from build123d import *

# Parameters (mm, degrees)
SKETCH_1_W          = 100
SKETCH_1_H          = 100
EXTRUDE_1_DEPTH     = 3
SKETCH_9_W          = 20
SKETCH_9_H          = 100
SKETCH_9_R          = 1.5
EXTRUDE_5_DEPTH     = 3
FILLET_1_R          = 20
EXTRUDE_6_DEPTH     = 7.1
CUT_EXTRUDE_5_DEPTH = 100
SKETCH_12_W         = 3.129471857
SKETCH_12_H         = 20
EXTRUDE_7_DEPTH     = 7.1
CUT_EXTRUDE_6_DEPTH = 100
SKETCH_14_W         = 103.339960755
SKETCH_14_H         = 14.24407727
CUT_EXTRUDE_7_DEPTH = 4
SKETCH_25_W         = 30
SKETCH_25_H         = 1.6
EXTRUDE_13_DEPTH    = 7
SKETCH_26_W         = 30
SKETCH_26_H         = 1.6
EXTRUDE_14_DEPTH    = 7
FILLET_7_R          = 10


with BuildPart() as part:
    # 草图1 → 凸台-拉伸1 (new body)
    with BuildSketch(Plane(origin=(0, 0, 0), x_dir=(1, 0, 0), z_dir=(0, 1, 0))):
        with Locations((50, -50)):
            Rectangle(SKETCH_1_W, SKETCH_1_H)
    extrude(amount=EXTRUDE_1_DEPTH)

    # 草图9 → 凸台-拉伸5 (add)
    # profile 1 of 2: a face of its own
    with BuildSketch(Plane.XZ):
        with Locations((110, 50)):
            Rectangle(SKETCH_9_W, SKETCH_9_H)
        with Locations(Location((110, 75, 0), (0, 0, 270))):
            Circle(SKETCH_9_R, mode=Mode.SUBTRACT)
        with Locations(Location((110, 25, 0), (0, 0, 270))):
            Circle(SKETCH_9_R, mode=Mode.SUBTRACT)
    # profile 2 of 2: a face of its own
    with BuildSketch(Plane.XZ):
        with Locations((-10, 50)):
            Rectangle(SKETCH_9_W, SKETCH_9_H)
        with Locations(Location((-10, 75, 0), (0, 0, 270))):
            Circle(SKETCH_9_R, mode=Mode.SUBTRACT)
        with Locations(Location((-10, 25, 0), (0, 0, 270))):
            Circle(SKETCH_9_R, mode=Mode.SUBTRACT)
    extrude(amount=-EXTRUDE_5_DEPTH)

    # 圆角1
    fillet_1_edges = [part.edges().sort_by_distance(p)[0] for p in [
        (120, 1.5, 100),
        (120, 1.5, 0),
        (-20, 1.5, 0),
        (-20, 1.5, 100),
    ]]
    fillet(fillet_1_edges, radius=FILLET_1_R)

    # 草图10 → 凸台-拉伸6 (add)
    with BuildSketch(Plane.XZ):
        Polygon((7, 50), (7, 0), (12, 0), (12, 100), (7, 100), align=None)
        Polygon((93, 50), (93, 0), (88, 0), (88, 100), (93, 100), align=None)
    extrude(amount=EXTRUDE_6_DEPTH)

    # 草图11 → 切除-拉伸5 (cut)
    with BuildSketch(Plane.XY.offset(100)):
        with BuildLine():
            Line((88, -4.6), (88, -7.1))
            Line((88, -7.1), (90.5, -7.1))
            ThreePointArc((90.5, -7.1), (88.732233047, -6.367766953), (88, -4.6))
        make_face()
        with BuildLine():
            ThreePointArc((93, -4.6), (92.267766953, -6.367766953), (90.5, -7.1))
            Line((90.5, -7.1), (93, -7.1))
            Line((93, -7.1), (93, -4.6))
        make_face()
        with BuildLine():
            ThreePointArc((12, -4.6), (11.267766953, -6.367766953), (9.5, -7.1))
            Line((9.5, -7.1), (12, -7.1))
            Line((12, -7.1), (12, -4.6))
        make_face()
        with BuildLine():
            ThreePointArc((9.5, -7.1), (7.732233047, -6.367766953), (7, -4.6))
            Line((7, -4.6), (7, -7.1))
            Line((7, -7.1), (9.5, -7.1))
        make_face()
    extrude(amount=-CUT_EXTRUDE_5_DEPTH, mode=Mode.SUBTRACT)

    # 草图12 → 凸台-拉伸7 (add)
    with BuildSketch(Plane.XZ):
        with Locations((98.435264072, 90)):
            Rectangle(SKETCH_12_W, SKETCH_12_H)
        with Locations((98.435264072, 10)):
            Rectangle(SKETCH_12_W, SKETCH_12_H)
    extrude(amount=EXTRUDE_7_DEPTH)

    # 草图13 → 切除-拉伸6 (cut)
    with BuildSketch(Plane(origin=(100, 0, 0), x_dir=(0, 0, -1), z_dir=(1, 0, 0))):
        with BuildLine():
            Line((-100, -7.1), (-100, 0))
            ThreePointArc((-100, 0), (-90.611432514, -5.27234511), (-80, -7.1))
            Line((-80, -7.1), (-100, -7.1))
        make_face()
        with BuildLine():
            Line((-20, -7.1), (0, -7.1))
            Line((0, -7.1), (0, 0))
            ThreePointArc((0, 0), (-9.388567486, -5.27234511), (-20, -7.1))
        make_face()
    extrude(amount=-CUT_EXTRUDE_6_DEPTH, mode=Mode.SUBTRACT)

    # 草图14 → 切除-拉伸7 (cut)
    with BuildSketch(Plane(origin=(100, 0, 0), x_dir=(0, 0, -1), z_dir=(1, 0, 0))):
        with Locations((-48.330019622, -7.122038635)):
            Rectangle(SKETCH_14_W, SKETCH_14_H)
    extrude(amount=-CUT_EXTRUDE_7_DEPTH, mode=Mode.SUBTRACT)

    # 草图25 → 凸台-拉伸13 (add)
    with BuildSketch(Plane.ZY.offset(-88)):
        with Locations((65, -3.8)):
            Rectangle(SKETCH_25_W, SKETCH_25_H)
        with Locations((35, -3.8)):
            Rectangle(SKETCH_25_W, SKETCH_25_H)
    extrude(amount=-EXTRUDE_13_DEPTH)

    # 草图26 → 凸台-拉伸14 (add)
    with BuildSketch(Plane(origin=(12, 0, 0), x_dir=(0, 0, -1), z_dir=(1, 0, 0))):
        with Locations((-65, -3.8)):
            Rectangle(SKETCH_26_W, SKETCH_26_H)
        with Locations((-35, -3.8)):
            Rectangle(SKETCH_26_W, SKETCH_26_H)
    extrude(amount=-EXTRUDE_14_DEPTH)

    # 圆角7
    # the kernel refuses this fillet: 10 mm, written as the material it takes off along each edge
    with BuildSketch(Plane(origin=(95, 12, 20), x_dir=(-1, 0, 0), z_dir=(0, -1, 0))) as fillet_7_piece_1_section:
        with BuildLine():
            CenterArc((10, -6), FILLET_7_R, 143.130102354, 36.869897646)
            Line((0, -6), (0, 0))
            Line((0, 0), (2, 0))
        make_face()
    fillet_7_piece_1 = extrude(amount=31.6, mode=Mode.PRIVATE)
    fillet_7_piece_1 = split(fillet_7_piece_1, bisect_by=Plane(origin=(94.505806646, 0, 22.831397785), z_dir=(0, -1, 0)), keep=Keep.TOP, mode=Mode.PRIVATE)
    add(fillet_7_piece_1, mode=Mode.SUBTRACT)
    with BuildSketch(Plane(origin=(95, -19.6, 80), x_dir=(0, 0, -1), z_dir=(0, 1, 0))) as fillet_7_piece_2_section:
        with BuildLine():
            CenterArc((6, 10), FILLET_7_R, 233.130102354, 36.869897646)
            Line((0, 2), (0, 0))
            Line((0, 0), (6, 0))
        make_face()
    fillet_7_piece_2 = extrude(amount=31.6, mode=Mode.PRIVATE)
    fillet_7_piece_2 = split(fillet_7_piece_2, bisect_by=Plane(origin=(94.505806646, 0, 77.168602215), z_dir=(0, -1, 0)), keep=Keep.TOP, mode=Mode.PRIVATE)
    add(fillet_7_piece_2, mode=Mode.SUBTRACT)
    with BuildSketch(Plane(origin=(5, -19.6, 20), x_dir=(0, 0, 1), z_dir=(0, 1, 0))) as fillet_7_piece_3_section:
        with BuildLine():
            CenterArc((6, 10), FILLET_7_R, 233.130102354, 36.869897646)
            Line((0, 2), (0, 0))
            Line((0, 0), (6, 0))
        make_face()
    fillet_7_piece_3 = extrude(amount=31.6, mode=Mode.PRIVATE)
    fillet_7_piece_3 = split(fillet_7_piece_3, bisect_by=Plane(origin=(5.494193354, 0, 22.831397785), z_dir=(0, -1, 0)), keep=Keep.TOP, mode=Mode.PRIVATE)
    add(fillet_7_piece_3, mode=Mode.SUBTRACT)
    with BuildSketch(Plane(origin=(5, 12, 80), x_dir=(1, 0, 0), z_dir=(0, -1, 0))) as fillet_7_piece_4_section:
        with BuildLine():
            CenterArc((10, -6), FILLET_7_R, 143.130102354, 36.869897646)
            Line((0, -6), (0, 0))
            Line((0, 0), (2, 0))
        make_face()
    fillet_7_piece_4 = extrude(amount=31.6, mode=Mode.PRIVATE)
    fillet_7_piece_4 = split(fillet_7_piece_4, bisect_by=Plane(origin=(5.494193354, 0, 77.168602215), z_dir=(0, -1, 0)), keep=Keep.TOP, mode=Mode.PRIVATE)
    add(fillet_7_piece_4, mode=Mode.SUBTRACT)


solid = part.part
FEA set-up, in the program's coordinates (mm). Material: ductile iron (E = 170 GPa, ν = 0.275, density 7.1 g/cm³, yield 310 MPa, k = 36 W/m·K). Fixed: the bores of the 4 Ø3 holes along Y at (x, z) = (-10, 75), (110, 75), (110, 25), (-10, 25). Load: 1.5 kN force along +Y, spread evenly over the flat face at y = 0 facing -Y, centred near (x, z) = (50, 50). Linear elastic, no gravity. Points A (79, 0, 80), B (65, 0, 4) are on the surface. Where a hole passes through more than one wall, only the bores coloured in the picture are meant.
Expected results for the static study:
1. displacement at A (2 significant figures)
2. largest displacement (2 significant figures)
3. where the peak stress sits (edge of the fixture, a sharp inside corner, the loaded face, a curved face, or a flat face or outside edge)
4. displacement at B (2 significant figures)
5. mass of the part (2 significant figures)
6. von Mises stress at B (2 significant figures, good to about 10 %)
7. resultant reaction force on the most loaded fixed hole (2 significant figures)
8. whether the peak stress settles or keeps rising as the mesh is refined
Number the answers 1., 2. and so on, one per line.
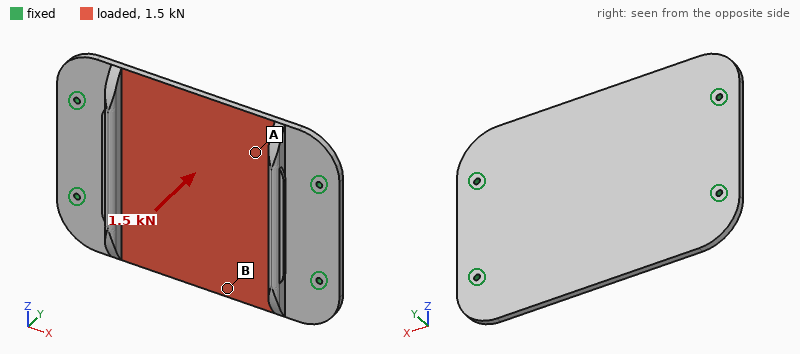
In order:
1. 0.22 mm
2. 0.36 mm
3. edge of the fixture
4. 0.31 mm
5. 330 g
6. 74 MPa
7. 380 N
8. keeps rising
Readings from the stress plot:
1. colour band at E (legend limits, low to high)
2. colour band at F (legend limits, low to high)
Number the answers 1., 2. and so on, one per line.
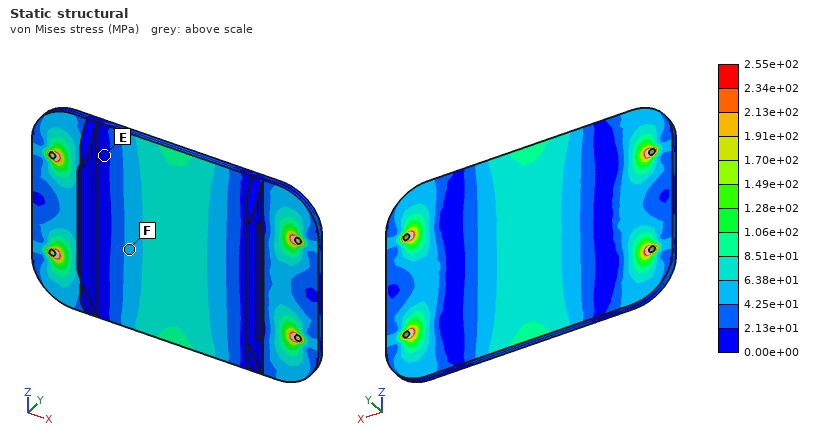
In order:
1. 0.00e+00 to 2.13e+01 MPa
2. 4.25e+01 to 6.38e+01 MPa
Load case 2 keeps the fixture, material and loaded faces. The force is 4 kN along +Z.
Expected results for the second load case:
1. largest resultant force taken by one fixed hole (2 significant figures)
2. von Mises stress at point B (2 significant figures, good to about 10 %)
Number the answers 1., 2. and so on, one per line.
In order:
1. 1.1 kN
2. 7.8 MPa
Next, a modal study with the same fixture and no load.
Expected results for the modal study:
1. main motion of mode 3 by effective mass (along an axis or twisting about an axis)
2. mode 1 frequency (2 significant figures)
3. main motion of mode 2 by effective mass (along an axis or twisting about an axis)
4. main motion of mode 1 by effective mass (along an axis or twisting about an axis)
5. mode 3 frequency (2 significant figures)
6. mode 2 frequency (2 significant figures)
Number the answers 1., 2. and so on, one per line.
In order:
1. twisting about Z
2. 870 Hz
3. twisting about X
4. along Y
5. 2300 Hz
6. 1200 Hz
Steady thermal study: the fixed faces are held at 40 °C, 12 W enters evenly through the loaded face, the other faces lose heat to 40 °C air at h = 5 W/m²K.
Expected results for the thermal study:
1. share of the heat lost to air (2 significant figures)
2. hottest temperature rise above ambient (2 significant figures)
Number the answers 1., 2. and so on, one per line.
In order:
1. 15 %
2. 26 K
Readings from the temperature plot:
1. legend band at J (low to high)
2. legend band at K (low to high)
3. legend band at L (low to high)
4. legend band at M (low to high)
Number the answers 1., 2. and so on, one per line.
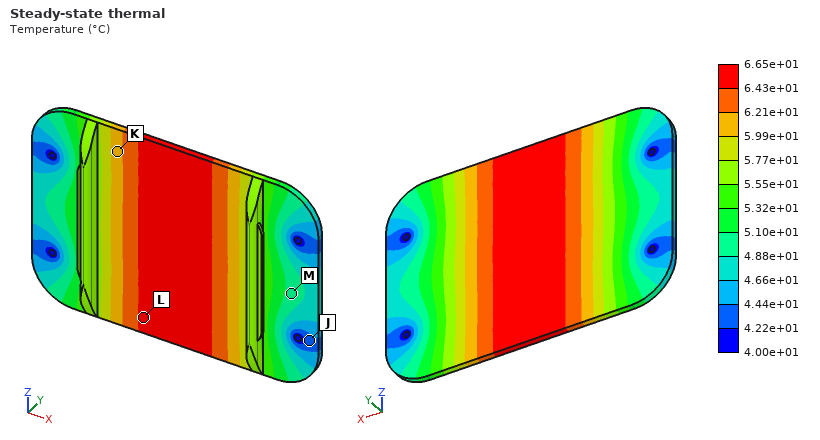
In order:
1. 4.22e+01 to 4.44e+01 °C
2. 5.99e+01 to 6.21e+01 °C
3. 6.43e+01 to 6.65e+01 °C
4. 4.88e+01 to 5.10e+01 °C
